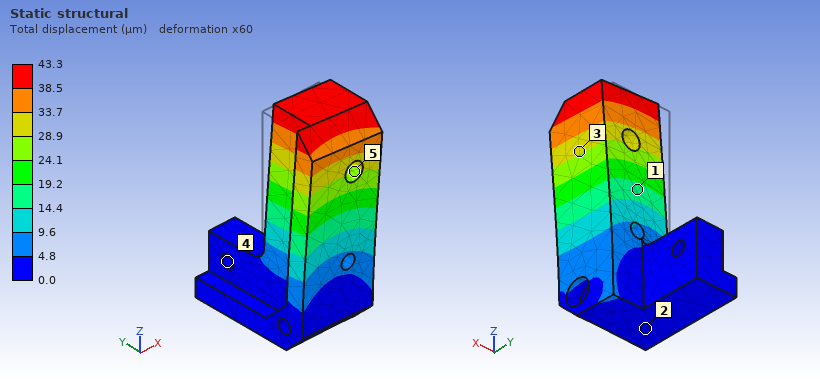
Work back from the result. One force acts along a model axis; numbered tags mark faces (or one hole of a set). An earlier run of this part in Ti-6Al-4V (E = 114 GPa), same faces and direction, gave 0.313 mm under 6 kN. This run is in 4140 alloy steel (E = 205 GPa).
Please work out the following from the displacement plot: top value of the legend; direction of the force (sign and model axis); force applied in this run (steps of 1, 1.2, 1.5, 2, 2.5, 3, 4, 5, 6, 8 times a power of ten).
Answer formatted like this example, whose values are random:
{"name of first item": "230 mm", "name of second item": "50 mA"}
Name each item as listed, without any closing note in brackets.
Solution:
{"top value of the legend": "43.3 µm", "direction of the force": "+X", "force applied in this run": "1.5 kN"}
